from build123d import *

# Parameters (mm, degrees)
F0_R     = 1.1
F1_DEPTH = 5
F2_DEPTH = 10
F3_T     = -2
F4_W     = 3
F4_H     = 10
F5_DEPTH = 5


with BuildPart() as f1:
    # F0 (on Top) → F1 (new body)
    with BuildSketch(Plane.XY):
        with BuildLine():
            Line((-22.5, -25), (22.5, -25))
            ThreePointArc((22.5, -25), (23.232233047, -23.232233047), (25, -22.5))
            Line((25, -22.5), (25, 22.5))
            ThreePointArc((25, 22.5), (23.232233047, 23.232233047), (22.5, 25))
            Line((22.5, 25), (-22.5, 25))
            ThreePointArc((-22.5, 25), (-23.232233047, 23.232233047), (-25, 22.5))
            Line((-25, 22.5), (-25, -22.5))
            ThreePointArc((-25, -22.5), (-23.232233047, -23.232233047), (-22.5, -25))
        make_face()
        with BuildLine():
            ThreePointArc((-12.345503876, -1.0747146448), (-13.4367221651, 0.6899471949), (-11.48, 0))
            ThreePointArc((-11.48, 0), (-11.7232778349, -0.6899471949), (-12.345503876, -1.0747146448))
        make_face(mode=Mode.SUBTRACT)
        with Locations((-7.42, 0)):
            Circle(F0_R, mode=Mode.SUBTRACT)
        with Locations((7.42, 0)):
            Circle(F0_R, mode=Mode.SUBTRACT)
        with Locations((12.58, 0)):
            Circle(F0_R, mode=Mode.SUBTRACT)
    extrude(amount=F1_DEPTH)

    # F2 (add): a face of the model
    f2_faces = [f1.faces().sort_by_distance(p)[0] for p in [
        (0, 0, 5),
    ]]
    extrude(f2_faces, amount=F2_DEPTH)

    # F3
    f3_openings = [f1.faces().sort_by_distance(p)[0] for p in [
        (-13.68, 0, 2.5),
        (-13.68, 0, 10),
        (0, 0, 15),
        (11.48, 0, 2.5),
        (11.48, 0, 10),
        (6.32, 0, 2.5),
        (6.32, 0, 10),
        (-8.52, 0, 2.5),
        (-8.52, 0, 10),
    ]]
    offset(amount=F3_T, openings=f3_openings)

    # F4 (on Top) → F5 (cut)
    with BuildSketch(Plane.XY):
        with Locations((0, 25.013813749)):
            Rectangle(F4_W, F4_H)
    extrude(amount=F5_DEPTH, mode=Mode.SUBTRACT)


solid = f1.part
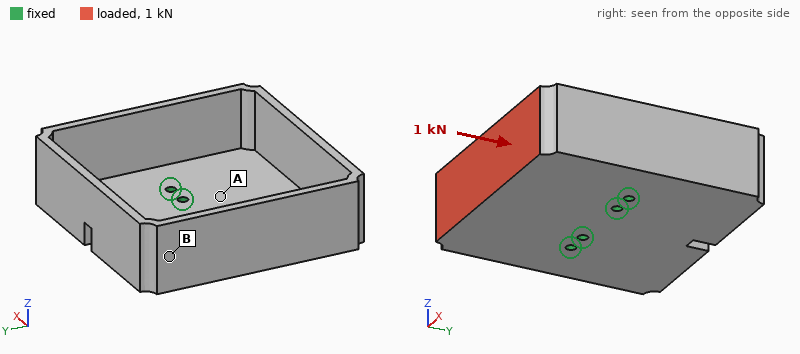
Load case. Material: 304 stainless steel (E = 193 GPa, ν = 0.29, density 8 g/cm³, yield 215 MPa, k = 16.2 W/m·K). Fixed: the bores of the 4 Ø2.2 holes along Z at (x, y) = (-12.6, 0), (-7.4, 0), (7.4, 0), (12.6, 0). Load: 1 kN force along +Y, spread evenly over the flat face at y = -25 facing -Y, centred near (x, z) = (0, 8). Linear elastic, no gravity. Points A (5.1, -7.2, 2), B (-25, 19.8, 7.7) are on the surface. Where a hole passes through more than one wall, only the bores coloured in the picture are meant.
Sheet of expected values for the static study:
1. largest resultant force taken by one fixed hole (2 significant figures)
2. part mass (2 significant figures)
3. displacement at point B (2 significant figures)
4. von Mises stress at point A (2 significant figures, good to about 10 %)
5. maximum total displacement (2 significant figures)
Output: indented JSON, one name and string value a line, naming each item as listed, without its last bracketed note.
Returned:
{
  "largest resultant force taken by one fixed hole": "320 N",
  "part mass": "78 g",
  "displacement at point B": "0.083 mm",
  "von Mises stress at point A": "75 MPa",
  "maximum total displacement": "0.18 mm"
}
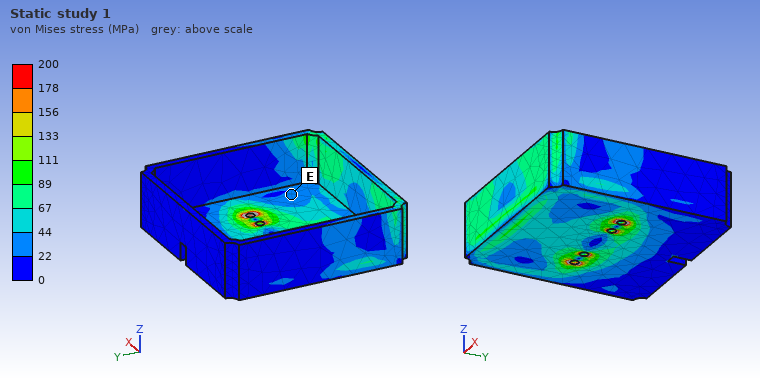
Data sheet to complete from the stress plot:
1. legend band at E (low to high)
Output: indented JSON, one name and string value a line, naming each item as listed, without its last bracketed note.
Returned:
{
  "legend band at E": "22 to 44 MPa"
}
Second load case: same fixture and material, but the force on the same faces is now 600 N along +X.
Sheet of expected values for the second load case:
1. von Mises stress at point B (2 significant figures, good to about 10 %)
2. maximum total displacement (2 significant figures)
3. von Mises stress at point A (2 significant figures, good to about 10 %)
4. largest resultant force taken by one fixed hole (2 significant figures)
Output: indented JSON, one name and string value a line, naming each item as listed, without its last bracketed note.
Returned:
{
  "von Mises stress at point B": "15 MPa",
  "maximum total displacement": "60 µm",
  "von Mises stress at point A": "43 MPa",
  "largest resultant force taken by one fixed hole": "520 N"
}
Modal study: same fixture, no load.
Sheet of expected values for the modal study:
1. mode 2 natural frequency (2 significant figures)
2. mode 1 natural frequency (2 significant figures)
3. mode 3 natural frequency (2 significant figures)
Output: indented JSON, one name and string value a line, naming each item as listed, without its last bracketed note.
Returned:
{
  "mode 2 natural frequency": "2200 Hz",
  "mode 1 natural frequency": "1300 Hz",
  "mode 3 natural frequency": "2900 Hz"
}
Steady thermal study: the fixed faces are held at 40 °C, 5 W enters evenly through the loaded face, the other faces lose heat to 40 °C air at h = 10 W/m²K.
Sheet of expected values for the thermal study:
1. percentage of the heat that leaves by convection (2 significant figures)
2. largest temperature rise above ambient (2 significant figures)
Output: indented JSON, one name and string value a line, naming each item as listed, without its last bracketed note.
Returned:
{
  "percentage of the heat that leaves by convection": "36 %",
  "largest temperature rise above ambient": "65 K"
}
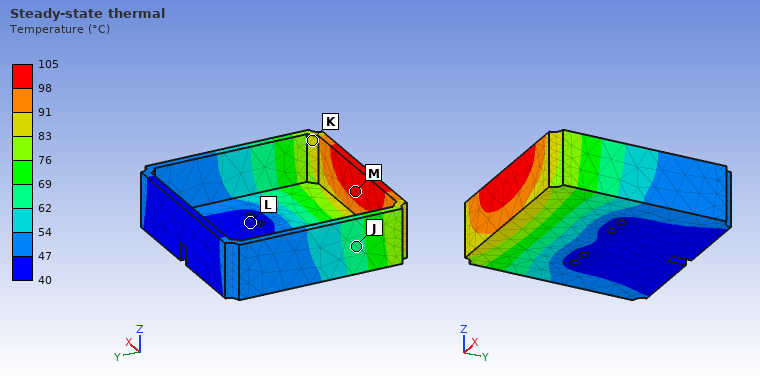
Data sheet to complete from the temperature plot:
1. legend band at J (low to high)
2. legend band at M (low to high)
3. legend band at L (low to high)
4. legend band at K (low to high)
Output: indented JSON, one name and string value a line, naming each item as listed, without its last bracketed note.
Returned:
{
  "legend band at J": "62 to 69 °C",
  "legend band at M": "98 to 105 °C",
  "legend band at L": "40 to 47 °C",
  "legend band at K": "83 to 91 °C"
}
